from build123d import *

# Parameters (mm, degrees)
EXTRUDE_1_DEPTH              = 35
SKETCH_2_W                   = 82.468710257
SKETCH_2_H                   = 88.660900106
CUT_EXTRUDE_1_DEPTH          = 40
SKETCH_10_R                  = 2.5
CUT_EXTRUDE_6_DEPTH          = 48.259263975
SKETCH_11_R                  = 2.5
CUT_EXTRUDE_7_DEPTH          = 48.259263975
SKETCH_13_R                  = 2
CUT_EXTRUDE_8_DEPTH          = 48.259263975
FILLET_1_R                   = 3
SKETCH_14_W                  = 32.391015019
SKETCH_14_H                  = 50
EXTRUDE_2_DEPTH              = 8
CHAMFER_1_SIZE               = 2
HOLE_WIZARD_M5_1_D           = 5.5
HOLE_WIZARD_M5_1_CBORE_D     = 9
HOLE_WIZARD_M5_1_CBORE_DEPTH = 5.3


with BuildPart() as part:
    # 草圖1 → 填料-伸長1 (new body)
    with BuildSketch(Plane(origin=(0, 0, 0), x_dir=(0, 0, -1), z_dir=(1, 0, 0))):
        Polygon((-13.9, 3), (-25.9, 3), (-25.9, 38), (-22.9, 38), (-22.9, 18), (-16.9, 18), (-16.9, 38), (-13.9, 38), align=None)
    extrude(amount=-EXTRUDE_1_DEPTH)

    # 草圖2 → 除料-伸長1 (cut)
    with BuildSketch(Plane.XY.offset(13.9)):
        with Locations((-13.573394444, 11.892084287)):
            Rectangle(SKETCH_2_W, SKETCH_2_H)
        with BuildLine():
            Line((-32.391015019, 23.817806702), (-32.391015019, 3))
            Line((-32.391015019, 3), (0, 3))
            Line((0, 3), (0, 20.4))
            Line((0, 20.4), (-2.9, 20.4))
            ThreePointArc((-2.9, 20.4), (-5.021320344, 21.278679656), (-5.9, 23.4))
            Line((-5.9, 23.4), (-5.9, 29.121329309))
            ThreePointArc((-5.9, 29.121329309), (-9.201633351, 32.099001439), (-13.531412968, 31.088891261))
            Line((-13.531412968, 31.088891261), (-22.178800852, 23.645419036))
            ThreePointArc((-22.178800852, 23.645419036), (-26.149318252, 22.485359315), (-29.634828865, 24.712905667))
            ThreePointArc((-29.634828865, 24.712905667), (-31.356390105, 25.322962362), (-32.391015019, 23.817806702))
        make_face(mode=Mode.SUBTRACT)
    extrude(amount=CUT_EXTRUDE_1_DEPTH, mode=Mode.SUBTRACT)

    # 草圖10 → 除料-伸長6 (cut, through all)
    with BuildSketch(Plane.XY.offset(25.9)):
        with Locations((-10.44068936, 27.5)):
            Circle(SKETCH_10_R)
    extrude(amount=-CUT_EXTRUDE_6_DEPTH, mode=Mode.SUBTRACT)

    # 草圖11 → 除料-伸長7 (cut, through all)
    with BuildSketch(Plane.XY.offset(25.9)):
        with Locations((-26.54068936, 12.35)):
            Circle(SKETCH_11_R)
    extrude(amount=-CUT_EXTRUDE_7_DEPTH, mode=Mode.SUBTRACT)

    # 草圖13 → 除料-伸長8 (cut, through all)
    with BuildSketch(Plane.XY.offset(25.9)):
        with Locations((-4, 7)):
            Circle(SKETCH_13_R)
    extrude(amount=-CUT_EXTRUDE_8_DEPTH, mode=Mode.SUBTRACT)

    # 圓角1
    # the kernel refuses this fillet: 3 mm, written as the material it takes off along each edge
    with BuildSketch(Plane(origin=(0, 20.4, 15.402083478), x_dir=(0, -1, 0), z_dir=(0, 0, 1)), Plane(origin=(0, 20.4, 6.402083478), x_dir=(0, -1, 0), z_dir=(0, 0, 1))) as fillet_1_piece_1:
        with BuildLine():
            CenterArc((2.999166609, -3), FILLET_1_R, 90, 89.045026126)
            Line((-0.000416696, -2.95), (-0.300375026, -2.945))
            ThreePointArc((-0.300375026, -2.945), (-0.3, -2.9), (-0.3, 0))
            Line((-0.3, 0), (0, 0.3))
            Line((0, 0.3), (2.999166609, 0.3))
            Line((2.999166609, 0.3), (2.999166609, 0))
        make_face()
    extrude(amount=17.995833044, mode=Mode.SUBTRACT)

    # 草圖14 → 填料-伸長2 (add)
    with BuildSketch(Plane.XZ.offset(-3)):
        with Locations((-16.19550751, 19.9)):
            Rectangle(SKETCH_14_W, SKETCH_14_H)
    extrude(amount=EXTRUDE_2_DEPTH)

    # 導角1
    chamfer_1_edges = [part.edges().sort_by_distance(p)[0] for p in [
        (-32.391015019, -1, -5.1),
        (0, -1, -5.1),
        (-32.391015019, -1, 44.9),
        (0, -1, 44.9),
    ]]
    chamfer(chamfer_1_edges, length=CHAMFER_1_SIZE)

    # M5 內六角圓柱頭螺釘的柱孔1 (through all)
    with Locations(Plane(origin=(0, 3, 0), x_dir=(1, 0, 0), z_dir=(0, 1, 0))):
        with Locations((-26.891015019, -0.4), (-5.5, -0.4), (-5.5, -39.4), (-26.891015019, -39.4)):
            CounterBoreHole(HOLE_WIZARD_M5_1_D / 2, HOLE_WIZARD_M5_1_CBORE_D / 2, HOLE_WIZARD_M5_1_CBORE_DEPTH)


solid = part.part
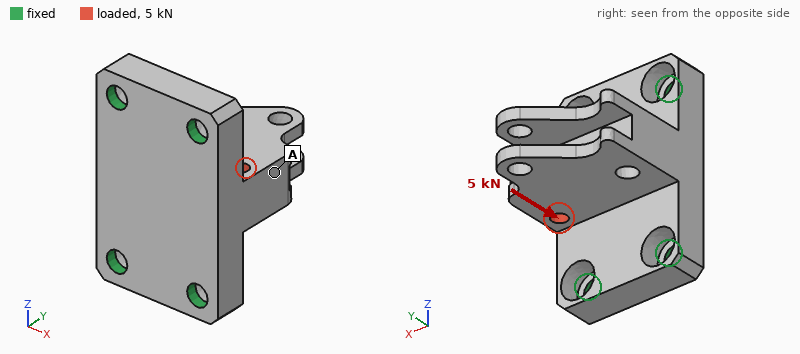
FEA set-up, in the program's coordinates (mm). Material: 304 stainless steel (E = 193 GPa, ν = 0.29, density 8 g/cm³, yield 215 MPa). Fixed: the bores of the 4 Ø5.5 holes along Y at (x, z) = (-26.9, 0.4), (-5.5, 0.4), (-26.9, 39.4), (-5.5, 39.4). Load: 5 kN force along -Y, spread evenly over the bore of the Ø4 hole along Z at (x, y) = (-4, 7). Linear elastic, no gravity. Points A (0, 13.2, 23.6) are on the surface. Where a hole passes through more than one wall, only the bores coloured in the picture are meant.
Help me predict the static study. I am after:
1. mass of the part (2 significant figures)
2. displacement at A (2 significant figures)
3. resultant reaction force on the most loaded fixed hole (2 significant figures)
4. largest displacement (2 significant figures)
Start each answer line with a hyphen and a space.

- 150 g
- 24 µm
- 3.5 kN
- 29 µm
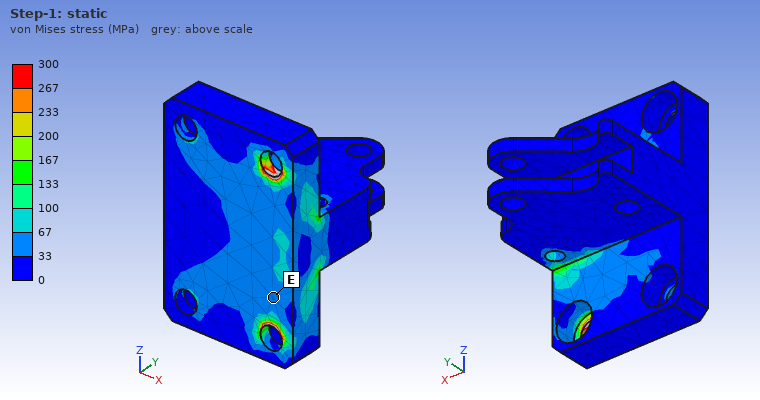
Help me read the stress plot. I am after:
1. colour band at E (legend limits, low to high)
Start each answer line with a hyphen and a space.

- 33 to 67 MPa
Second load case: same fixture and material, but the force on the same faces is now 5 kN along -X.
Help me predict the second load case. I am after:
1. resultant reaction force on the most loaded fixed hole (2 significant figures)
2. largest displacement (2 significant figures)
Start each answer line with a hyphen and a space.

- 2.2 kN
- 22 µm
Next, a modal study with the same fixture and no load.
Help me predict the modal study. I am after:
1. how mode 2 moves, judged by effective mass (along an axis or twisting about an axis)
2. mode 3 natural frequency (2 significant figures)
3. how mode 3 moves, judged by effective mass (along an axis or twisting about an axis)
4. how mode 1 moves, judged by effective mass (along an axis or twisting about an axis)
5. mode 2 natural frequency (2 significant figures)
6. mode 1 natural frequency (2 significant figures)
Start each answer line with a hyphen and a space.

- along Z
- 12 kHz
- along Y
- along X
- 10 kHz
- 9100 Hz
